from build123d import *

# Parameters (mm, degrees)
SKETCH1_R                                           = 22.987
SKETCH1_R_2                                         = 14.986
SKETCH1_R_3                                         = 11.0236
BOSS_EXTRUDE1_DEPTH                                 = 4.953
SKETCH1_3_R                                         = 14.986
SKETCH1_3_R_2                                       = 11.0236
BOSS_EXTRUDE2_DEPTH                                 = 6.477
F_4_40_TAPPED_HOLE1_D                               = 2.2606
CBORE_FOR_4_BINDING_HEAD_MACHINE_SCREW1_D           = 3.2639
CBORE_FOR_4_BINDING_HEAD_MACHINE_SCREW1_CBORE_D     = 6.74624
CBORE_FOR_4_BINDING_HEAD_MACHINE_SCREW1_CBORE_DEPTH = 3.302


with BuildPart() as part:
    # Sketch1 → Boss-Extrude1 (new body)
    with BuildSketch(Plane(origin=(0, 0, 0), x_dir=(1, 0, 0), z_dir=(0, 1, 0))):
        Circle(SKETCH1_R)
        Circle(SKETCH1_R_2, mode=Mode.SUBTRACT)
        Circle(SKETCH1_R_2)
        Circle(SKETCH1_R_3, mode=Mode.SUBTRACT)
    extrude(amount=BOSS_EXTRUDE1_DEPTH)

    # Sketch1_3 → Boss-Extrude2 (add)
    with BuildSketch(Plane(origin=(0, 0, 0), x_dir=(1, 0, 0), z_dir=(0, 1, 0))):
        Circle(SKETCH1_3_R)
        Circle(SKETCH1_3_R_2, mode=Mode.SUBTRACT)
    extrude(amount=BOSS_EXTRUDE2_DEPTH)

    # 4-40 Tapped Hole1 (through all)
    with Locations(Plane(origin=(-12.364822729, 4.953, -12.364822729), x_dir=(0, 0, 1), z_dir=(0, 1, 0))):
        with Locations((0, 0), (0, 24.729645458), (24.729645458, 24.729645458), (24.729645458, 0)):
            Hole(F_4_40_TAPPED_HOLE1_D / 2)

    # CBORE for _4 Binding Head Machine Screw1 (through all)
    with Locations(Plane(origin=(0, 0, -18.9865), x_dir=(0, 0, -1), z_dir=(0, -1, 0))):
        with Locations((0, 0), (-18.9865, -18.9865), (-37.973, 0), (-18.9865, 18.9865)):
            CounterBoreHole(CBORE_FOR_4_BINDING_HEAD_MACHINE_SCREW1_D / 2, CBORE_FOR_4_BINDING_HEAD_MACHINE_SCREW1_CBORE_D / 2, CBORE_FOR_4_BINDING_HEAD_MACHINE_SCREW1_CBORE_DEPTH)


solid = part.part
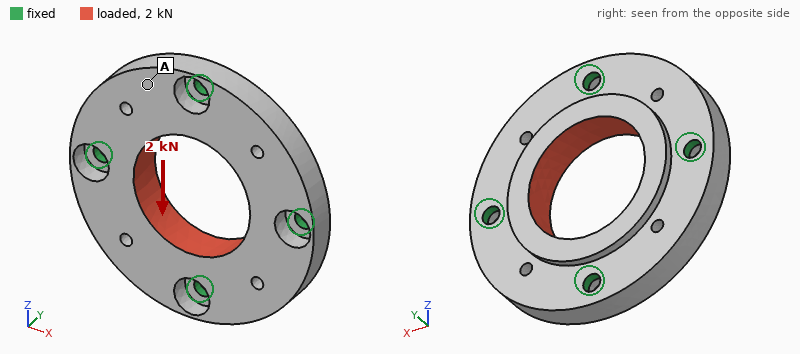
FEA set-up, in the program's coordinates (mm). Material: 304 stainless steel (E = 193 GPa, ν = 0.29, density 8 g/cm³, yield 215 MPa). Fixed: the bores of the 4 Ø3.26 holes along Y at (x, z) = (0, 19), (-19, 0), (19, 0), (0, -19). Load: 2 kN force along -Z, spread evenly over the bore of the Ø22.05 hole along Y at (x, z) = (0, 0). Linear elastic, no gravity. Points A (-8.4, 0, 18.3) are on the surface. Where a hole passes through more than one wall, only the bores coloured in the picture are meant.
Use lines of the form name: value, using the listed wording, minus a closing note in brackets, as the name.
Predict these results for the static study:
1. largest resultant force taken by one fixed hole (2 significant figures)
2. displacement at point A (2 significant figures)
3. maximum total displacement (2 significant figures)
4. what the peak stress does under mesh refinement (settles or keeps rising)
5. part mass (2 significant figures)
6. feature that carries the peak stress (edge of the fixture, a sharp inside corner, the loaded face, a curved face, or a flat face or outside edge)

largest resultant force taken by one fixed hole: 520 N
displacement at point A: 1.1 µm
maximum total displacement: 1.2 µm
what the peak stress does under mesh refinement: keeps rising
part mass: 50 g
feature that carries the peak stress: edge of the fixture
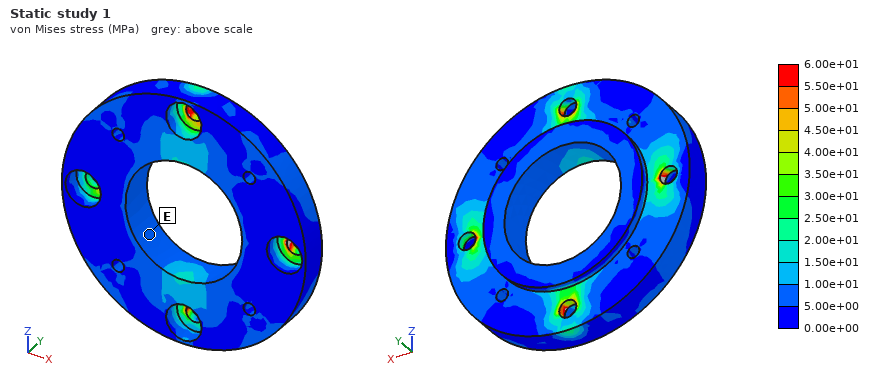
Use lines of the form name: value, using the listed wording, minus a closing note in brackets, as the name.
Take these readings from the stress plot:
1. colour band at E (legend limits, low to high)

colour band at E: 5.00e+00 to 1.00e+01 MPa
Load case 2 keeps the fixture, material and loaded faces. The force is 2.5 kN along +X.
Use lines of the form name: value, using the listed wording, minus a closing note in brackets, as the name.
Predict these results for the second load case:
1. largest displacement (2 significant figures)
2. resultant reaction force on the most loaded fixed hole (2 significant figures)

largest displacement: 1.6 µm
resultant reaction force on the most loaded fixed hole: 650 N
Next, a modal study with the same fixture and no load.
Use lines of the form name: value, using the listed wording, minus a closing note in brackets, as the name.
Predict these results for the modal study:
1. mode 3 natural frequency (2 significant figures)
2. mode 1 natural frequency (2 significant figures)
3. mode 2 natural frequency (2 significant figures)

mode 3 natural frequency: 17 kHz
mode 1 natural frequency: 14 kHz
mode 2 natural frequency: 17 kHz
